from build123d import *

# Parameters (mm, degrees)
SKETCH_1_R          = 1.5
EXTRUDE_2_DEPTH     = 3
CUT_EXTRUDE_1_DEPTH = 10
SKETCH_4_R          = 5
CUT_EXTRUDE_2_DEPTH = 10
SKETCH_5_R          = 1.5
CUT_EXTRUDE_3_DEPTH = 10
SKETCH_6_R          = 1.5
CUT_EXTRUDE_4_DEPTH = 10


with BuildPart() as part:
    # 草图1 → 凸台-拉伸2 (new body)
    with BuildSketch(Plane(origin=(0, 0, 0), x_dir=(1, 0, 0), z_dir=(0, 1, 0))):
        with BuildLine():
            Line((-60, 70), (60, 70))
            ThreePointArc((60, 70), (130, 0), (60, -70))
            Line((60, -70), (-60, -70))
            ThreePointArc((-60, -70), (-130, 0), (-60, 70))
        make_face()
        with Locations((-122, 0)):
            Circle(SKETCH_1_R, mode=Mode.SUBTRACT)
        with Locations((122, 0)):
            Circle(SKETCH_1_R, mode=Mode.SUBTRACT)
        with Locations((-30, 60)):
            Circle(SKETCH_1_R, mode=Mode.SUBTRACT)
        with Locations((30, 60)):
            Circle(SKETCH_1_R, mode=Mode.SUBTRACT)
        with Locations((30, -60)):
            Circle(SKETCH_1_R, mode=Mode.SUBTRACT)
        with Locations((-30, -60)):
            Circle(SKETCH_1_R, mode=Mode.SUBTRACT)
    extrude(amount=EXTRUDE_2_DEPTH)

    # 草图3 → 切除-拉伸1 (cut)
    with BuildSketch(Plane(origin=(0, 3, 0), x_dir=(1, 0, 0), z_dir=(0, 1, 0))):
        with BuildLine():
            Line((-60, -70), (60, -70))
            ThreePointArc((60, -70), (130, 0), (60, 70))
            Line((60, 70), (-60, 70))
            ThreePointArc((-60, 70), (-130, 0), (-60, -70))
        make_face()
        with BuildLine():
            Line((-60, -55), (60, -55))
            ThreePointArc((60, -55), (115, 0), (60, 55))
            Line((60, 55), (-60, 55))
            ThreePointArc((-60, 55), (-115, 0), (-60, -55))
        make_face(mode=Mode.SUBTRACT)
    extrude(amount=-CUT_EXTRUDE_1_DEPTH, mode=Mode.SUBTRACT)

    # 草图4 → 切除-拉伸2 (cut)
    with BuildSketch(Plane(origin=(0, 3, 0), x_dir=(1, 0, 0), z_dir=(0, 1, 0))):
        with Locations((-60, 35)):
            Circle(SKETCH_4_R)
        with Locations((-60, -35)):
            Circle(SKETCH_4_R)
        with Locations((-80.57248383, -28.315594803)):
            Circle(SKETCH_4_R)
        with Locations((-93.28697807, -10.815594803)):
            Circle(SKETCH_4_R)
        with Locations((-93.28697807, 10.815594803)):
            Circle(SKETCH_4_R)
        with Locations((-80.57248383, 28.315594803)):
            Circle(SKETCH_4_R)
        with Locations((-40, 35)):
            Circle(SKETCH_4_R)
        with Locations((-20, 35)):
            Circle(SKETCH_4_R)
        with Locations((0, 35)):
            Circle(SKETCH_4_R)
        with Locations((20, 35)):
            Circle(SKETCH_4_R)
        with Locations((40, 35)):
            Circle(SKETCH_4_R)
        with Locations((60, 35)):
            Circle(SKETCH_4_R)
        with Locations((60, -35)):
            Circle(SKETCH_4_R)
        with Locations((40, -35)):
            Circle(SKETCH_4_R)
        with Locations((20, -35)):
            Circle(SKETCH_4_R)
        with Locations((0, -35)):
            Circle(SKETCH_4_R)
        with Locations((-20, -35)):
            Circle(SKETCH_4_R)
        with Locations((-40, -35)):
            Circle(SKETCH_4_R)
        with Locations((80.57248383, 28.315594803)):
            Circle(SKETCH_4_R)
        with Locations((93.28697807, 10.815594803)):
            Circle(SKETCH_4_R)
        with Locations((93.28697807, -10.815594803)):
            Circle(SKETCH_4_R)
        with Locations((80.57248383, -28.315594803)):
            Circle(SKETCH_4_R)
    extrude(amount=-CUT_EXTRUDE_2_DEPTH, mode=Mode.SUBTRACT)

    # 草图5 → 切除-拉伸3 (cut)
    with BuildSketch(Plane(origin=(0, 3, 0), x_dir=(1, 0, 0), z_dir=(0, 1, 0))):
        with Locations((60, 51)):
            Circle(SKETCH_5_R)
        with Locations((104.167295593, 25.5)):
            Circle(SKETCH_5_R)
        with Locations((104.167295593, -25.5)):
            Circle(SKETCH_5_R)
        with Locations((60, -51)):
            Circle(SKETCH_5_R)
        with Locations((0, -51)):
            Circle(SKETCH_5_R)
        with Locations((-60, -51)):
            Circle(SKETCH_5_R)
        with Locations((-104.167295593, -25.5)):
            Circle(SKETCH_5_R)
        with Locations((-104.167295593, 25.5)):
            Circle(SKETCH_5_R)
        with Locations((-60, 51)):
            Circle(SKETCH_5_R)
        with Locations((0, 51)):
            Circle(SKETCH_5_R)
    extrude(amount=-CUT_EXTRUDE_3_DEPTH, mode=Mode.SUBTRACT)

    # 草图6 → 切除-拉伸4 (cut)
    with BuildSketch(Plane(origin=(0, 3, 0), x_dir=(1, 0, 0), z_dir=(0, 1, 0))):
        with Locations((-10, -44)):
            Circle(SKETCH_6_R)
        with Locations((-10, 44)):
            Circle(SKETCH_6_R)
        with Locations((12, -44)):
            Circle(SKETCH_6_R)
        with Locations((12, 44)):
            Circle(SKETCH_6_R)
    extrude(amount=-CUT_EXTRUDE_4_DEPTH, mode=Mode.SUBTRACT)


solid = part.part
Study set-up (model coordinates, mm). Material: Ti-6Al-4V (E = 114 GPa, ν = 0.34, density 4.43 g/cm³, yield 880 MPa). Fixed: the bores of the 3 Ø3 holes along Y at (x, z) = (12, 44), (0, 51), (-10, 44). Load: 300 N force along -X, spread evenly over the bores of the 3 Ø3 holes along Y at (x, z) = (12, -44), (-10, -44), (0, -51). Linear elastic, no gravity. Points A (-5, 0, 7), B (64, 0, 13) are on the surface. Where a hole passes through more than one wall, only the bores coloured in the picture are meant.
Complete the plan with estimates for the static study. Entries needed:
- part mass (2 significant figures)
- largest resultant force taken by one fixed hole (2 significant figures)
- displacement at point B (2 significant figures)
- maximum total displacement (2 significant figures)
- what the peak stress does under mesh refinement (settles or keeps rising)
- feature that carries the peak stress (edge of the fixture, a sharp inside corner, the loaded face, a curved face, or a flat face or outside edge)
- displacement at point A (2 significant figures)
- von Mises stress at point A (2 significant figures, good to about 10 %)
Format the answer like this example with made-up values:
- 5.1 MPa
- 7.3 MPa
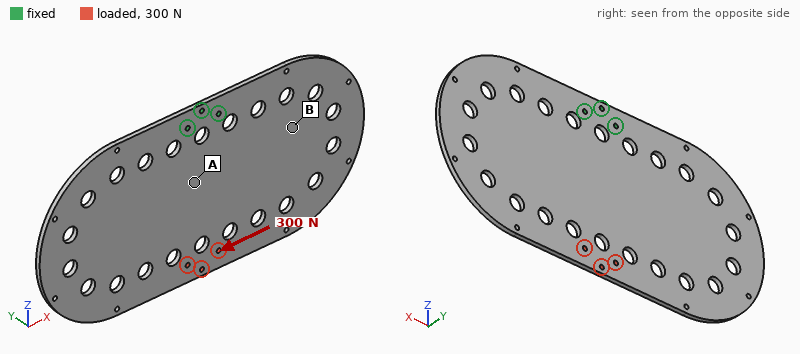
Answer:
- 280 g
- 1.1 kN
- 29 µm
- 55 µm
- keeps rising
- edge of the fixture
- 16 µm
- 5.9 MPa
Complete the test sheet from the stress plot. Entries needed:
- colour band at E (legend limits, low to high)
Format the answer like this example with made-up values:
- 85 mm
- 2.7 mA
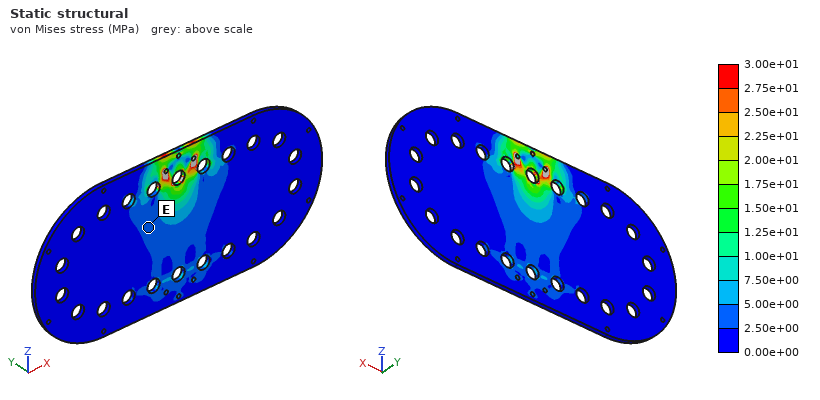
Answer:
- 2.50e+00 to 5.00e+00 MPa
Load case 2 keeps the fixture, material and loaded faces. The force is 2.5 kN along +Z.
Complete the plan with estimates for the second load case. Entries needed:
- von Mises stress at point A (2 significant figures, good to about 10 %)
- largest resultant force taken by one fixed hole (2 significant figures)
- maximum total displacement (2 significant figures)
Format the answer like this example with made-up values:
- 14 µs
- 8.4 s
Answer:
- 16 MPa
- 1.2 kN
- 20 µm
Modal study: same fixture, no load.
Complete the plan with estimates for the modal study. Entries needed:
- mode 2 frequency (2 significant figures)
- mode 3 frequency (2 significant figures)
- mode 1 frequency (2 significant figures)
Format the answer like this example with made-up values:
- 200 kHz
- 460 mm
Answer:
- 150 Hz
- 300 Hz
- 150 Hz
